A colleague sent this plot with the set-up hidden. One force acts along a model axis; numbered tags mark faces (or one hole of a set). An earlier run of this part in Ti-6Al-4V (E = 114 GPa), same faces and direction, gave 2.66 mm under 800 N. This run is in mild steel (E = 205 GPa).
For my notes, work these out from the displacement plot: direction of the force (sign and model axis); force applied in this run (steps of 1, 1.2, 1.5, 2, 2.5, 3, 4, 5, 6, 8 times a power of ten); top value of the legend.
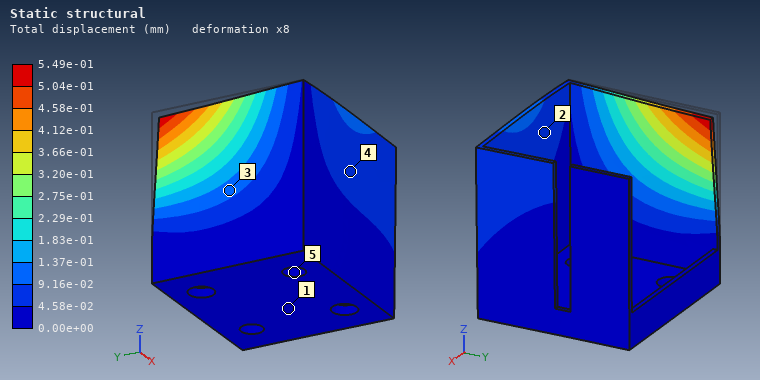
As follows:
+X
300 N
5.49e-01 mm
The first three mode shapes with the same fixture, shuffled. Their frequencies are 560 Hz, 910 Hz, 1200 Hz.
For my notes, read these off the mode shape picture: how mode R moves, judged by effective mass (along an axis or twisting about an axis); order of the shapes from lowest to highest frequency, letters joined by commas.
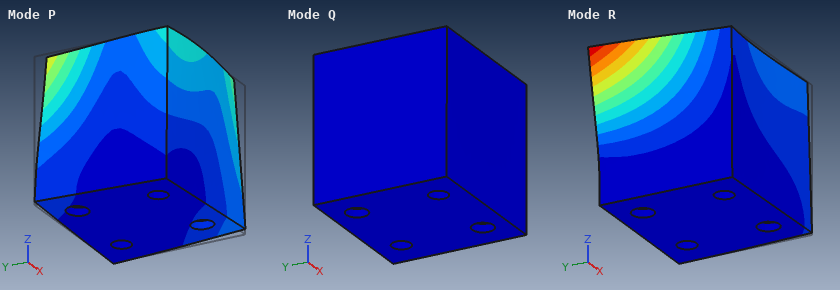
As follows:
along X
Q, R, P
